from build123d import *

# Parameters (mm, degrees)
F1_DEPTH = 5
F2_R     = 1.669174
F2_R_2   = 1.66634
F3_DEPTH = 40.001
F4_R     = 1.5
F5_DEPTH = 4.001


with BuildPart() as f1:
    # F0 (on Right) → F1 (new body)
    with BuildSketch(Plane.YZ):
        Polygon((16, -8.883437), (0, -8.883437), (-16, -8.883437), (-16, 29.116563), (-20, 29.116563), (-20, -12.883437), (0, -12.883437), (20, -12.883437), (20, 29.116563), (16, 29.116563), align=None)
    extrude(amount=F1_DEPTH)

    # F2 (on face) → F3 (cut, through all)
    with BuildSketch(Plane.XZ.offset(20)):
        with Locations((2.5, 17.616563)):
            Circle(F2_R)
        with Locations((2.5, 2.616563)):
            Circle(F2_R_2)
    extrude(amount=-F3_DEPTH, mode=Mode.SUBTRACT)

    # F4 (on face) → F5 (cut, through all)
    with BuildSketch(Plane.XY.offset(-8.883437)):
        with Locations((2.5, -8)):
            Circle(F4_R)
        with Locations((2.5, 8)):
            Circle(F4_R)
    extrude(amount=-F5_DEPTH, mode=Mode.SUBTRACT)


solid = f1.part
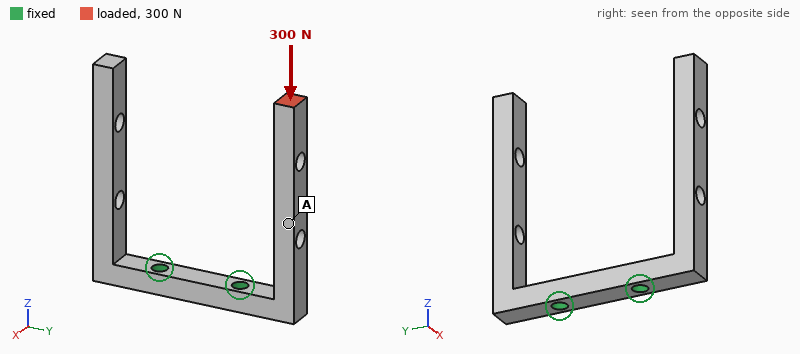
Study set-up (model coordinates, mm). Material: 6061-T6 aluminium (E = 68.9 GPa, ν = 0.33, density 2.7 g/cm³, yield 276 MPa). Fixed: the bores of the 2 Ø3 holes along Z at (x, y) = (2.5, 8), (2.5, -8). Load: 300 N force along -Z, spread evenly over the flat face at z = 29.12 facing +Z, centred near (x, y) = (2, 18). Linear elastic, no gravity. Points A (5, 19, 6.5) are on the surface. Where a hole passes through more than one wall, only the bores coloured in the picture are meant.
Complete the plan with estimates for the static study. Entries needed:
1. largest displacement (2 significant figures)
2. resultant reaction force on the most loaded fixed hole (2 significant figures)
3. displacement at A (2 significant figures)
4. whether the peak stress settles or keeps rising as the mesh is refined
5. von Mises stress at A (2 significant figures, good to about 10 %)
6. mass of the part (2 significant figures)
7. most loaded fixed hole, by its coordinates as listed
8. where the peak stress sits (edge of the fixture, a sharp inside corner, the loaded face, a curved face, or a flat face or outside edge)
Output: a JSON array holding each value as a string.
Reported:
["0.28 mm", "300 N", "0.13 mm", "keeps rising", "23 MPa", "5.7 g", "(2.5, 8)", "edge of the fixture"]
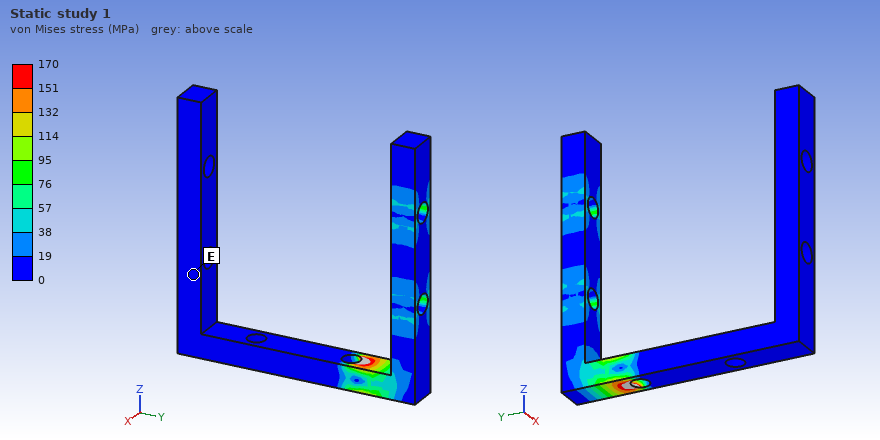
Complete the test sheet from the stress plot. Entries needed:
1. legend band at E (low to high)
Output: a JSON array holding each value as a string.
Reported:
["0 to 19 MPa"]
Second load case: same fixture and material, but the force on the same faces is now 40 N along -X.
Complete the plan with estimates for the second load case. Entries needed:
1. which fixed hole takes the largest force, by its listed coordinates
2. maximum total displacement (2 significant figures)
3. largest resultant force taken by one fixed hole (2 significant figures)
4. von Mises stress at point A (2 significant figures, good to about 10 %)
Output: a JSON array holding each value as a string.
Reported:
["(2.5, 8)", "0.66 mm", "42 N", "55 MPa"]
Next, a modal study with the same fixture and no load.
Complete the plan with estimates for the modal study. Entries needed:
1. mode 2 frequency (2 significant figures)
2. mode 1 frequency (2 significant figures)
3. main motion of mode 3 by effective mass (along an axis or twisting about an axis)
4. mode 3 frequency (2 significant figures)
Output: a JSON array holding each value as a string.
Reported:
["1500 Hz", "1500 Hz", "along X", "1600 Hz"]
